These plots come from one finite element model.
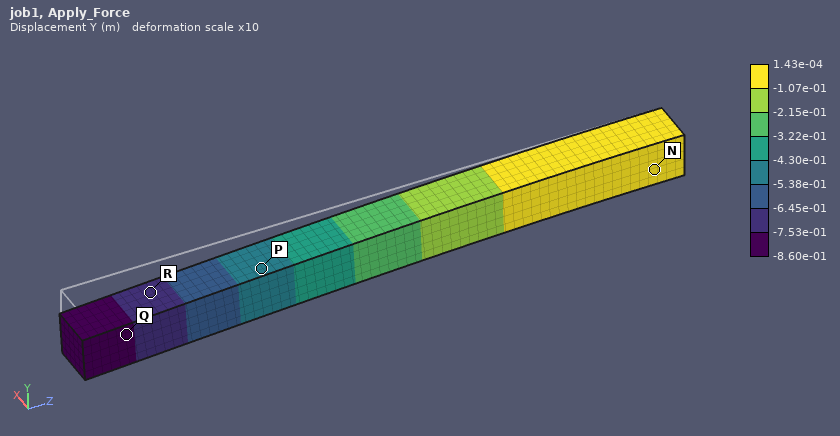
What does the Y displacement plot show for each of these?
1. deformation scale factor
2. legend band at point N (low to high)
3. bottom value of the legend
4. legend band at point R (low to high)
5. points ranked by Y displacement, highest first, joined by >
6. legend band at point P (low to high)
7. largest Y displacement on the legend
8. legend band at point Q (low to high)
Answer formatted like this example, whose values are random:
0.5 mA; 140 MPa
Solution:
10; -1.07e-01 to 1.43e-04 m; -8.60e-01 m; -7.53e-01 to -6.45e-01 m; N > P > R > Q; -5.38e-01 to -4.30e-01 m; 1.43e-04 m; -8.60e-01 to -7.53e-01 m
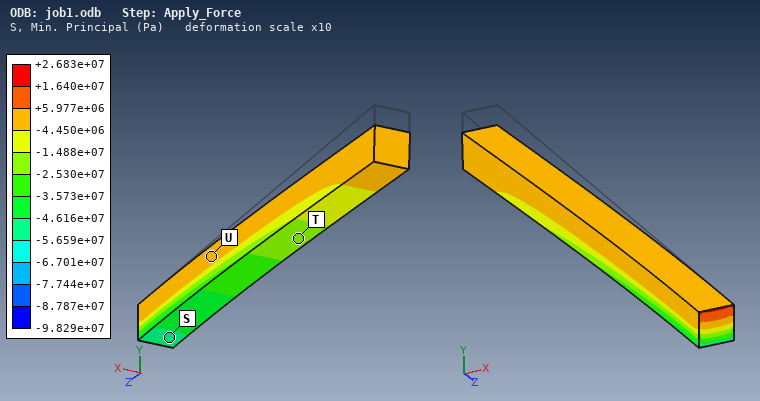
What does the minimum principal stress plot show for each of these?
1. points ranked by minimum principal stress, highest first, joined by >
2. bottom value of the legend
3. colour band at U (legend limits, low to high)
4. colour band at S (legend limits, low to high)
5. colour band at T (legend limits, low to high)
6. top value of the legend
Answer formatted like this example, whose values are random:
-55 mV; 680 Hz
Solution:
U > T > S; -9.829e+07 Pa; -4.450e+06 to +5.977e+06 Pa; -5.659e+07 to -4.616e+07 Pa; -2.530e+07 to -1.488e+07 Pa; +2.683e+07 Pa
